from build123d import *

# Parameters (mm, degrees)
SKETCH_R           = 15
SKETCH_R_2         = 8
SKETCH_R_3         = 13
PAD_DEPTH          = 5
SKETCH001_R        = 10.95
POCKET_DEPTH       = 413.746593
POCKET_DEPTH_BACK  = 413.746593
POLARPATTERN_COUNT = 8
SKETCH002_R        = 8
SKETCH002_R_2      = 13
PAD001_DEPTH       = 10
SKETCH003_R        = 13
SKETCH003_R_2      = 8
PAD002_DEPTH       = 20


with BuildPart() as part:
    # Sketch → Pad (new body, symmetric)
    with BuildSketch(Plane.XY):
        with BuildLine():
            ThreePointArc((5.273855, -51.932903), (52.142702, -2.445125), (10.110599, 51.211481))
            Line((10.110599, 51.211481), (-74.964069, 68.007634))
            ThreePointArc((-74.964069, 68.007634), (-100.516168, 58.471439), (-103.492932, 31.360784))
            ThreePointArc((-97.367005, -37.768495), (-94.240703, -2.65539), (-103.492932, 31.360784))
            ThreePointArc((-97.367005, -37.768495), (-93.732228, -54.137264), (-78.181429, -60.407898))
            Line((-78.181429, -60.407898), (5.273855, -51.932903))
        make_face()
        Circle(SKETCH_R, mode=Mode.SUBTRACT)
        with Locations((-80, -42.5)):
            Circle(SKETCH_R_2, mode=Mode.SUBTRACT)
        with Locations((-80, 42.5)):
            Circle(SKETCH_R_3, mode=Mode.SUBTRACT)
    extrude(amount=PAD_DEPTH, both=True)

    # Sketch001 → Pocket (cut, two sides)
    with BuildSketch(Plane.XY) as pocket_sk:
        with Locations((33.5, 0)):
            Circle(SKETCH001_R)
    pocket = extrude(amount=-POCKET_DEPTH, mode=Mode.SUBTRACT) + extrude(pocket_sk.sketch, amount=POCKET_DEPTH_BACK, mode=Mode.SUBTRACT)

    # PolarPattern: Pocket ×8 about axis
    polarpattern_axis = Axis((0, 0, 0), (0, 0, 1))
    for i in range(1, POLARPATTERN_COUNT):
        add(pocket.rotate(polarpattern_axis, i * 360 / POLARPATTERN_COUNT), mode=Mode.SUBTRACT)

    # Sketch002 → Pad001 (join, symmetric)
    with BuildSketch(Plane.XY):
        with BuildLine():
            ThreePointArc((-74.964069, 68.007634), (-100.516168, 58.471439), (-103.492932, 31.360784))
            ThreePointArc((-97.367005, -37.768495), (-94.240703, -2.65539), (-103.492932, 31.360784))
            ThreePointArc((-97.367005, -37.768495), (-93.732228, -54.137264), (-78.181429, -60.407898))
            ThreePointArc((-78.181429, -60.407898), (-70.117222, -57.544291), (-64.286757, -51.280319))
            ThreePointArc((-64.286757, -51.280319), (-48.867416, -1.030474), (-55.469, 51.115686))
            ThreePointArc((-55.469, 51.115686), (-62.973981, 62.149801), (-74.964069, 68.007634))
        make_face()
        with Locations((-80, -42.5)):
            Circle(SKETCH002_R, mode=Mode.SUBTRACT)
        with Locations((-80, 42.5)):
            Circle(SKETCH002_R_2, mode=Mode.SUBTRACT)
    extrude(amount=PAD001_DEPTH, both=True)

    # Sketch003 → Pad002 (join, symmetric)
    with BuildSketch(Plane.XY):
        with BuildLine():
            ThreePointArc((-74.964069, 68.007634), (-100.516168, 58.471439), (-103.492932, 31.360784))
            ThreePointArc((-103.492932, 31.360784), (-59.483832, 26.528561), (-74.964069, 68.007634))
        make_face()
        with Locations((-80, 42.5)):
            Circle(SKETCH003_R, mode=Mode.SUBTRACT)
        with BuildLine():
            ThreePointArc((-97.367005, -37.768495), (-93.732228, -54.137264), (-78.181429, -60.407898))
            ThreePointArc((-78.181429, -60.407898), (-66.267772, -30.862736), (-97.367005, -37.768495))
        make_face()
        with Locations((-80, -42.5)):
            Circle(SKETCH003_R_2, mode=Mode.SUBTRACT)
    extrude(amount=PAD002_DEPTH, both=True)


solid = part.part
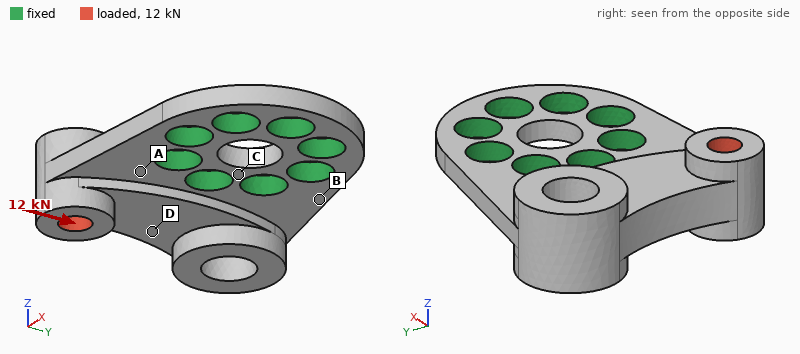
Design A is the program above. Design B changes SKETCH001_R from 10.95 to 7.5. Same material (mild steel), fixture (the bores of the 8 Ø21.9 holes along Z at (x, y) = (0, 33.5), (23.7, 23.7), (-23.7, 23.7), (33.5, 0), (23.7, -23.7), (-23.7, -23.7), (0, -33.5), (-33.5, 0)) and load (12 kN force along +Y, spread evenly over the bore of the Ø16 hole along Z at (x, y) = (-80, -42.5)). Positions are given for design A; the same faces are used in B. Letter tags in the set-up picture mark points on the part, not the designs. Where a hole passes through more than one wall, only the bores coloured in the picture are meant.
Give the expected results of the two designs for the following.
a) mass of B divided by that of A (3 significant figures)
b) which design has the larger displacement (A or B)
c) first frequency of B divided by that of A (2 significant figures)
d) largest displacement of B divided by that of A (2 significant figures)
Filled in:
1.08
B
0.86
1.2
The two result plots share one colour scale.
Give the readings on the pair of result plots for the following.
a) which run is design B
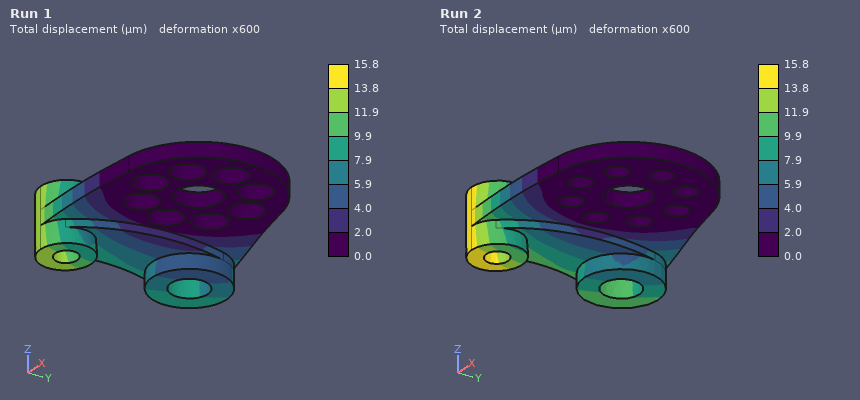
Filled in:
Run 2
